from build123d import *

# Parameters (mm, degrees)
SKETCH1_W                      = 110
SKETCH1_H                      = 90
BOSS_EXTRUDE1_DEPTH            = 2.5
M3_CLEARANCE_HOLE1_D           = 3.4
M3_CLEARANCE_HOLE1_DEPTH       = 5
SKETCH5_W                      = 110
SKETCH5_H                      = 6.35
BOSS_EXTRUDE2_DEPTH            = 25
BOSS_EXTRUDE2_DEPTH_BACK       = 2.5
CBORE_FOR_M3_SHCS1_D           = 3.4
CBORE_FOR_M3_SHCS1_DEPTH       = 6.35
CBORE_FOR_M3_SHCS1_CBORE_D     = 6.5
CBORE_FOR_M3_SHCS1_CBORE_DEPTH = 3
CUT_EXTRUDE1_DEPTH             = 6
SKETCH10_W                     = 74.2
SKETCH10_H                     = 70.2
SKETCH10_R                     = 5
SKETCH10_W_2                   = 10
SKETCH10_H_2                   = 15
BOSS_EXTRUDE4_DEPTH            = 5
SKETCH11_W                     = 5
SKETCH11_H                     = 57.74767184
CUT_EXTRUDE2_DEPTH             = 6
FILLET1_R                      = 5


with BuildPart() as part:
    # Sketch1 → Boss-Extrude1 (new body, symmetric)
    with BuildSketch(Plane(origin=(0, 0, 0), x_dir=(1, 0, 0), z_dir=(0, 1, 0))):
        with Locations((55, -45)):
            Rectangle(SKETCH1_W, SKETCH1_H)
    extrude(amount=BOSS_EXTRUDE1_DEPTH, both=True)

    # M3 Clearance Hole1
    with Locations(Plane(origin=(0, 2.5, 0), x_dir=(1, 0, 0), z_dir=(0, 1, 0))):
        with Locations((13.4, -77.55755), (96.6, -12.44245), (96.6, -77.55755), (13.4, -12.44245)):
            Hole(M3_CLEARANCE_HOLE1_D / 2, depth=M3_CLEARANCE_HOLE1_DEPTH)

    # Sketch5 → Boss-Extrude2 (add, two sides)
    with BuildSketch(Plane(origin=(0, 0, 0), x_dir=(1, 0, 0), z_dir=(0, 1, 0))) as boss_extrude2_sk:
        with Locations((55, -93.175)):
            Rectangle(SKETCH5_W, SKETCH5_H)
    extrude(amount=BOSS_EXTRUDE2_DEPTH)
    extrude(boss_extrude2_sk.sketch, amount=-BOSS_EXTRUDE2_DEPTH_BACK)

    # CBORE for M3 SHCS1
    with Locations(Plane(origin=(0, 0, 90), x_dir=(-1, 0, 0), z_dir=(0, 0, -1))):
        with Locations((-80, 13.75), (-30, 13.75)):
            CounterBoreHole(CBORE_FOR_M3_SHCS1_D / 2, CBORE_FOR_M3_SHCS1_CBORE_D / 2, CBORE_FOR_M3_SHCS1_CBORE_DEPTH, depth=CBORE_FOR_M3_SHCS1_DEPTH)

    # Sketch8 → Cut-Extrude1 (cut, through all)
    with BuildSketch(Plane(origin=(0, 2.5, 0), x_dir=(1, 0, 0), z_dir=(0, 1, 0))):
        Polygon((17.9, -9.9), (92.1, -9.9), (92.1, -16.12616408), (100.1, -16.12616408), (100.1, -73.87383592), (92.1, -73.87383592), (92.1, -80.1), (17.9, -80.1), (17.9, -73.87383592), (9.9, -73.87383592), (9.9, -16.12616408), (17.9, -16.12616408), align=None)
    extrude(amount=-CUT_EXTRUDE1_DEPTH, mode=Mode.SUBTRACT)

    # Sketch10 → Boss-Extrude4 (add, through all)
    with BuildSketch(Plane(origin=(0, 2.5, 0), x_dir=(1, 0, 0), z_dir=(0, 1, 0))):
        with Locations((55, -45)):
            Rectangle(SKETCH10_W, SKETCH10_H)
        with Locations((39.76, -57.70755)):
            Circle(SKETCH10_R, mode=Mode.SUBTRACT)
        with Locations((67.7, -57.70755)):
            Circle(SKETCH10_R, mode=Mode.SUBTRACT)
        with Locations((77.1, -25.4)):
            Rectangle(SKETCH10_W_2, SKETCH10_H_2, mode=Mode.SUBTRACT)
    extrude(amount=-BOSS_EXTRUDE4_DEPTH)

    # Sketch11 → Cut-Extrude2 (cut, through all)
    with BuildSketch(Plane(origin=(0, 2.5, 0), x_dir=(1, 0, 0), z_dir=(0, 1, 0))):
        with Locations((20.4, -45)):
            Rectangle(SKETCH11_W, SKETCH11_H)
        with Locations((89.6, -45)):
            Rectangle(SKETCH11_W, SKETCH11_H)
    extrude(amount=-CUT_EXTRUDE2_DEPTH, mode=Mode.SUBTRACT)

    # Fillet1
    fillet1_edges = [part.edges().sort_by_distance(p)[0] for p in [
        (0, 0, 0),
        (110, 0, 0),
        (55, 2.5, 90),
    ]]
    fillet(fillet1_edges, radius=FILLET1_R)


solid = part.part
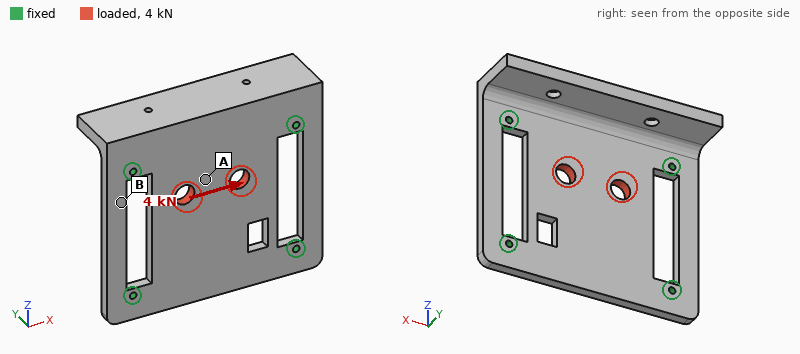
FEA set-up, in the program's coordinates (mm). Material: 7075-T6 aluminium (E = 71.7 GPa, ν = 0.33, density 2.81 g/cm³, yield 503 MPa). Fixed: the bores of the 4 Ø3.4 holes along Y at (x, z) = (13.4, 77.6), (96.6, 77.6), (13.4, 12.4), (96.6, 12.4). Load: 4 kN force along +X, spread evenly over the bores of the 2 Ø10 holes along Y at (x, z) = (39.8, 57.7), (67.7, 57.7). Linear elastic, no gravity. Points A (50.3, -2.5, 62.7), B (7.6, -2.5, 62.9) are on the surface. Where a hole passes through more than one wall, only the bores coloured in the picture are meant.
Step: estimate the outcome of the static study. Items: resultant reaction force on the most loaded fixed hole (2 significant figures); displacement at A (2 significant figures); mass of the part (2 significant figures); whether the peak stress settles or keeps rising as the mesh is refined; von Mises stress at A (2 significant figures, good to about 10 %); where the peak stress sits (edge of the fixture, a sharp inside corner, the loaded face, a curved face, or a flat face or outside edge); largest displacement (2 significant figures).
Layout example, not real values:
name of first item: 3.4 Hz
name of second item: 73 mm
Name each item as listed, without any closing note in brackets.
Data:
resultant reaction force on the most loaded fixed hole: 1.4 kN
displacement at A: 13 µm
mass of the part: 170 g
whether the peak stress settles or keeps rising as the mesh is refined: keeps rising
von Mises stress at A: 16 MPa
where the peak stress sits: edge of the fixture
largest displacement: 16 µm
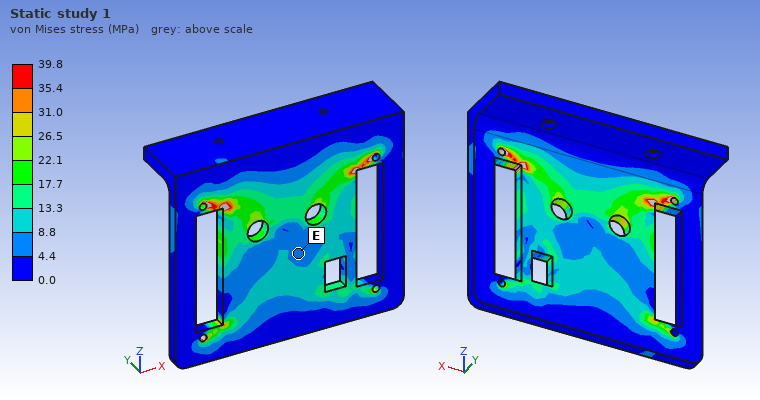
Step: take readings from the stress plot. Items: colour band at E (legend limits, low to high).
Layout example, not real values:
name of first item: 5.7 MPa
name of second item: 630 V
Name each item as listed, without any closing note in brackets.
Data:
colour band at E: 4.4 to 8.8 MPa
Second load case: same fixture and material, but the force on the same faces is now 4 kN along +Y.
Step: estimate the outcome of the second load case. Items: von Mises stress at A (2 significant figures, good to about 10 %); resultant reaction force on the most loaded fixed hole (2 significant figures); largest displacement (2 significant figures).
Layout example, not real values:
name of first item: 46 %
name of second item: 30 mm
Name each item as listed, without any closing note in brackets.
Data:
von Mises stress at A: 130 MPa
resultant reaction force on the most loaded fixed hole: 1.5 kN
largest displacement: 0.41 mm
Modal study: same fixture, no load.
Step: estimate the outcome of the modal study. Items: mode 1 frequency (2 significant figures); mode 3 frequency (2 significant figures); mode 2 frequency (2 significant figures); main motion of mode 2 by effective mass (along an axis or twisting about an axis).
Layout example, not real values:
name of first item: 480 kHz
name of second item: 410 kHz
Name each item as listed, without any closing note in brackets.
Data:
mode 1 frequency: 2200 Hz
mode 3 frequency: 4000 Hz
mode 2 frequency: 2900 Hz
main motion of mode 2 by effective mass: along Y
